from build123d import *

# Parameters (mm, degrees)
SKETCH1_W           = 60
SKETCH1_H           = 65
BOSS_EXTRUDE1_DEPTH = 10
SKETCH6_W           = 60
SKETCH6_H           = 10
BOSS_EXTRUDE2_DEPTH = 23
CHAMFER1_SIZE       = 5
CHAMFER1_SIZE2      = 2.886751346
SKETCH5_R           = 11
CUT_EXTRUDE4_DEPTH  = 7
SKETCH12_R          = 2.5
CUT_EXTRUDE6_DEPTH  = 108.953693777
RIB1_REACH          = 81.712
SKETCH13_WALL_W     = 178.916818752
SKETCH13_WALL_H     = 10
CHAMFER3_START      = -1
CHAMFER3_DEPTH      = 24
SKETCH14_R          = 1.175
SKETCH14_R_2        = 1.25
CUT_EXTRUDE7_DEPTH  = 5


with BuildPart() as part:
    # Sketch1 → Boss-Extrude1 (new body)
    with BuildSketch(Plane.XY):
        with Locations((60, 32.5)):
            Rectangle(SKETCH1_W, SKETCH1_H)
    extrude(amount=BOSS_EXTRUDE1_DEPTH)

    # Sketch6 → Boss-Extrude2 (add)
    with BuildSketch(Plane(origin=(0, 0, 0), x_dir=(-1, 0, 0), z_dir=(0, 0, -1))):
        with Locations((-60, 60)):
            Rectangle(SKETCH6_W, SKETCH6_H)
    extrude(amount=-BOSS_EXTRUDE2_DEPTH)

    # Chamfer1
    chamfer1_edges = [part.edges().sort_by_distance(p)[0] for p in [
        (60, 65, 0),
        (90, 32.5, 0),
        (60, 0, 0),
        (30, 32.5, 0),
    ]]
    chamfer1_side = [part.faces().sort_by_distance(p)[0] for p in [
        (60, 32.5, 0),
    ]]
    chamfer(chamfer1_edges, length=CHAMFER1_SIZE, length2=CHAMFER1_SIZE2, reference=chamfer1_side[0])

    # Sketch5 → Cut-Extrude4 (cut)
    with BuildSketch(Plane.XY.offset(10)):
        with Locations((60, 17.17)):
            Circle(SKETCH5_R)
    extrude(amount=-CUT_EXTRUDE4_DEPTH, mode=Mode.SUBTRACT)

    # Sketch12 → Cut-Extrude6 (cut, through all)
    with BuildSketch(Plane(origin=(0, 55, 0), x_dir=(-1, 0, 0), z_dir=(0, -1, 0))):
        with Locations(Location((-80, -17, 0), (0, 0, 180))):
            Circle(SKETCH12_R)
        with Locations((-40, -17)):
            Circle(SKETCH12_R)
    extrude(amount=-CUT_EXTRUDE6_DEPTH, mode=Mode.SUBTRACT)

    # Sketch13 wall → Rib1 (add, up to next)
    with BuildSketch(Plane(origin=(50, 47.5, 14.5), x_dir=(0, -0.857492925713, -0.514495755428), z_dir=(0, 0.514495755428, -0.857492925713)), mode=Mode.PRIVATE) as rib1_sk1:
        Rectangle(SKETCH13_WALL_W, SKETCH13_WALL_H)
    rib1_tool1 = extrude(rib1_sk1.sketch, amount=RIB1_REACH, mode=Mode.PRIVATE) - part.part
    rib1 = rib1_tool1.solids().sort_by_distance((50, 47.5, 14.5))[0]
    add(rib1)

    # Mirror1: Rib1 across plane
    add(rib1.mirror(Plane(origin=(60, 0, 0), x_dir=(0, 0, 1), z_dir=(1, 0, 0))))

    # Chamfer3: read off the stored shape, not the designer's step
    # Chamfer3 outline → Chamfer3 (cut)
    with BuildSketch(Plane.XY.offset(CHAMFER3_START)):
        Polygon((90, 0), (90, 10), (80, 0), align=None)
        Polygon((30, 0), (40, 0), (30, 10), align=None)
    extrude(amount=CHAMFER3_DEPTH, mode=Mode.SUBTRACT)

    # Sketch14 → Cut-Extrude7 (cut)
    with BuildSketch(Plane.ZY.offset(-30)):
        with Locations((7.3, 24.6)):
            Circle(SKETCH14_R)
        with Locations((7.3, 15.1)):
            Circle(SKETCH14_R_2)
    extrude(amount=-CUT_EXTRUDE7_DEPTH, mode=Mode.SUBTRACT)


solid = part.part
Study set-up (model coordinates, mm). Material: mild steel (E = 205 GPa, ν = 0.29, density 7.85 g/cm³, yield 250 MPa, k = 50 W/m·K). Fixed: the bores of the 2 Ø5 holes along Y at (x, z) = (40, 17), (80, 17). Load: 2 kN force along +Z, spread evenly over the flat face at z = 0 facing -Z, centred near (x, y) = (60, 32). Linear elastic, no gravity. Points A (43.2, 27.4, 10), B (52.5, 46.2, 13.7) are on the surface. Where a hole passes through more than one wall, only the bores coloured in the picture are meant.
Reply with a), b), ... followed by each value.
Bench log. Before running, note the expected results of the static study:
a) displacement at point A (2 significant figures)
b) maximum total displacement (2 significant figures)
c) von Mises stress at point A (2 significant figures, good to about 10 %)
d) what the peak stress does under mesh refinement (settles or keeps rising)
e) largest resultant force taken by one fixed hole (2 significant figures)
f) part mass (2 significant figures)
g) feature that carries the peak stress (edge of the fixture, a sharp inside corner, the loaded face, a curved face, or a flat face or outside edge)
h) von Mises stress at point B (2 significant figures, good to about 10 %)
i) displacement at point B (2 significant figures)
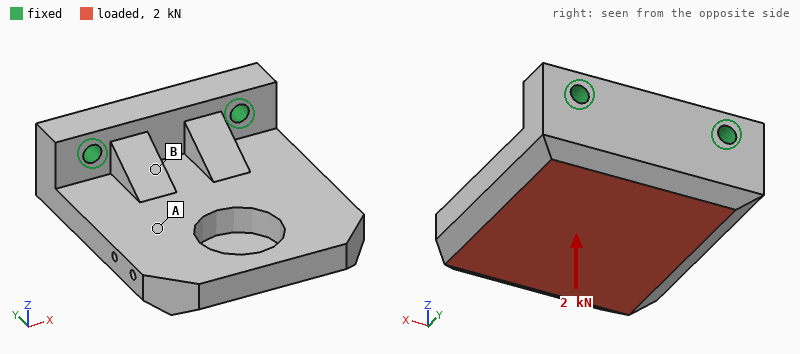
a) 29 µm
b) 65 µm
c) 13 MPa
d) keeps rising
e) 1.1 kN
f) 330 g
g) edge of the fixture
h) 33 MPa
i) 10 µm
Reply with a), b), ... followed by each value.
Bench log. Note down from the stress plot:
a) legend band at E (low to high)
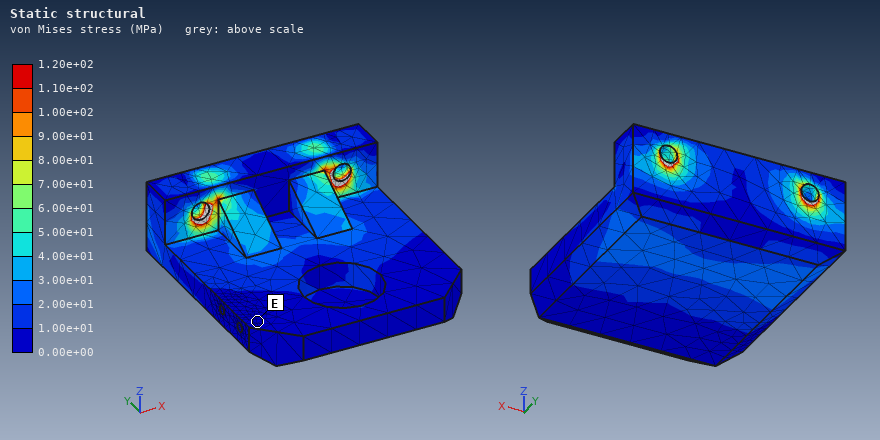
a) 0.00e+00 to 1.00e+01 MPa
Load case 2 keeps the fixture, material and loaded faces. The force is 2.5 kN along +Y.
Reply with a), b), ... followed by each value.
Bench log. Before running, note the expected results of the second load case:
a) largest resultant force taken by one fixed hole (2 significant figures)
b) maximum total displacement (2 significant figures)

a) 1.3 kN
b) 35 µm
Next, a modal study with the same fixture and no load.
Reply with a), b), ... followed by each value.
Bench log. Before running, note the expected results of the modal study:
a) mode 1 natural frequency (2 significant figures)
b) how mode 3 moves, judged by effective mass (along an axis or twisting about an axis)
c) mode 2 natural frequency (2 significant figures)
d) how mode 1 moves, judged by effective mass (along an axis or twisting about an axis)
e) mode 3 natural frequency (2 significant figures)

a) 2200 Hz
b) along X
c) 5000 Hz
d) along Z
e) 6800 Hz
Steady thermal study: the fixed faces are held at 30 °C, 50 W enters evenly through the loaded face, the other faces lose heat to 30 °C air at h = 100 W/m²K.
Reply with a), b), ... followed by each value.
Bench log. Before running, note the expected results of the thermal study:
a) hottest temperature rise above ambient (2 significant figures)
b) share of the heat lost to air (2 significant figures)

a) 39 K
b) 39 %
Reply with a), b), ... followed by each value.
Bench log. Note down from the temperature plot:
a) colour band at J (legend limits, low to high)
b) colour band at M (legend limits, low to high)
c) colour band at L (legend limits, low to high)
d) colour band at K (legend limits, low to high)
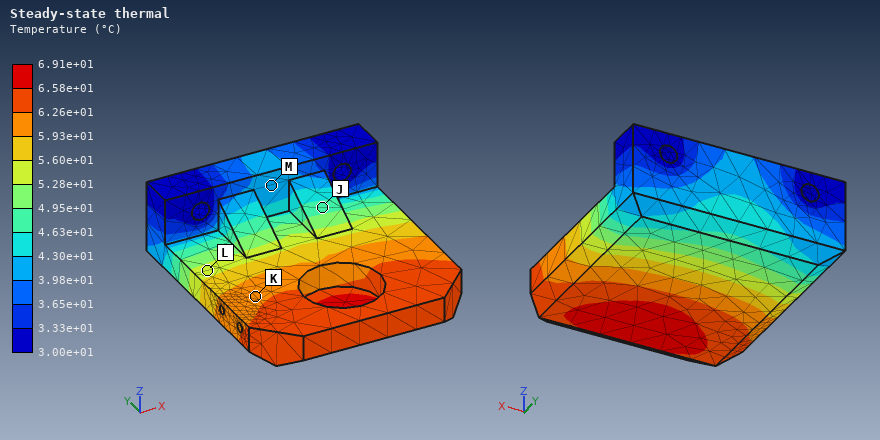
a) 4.63e+01 to 4.95e+01 °C
b) 3.98e+01 to 4.30e+01 °C
c) 5.28e+01 to 5.60e+01 °C
d) 5.93e+01 to 6.26e+01 °C
